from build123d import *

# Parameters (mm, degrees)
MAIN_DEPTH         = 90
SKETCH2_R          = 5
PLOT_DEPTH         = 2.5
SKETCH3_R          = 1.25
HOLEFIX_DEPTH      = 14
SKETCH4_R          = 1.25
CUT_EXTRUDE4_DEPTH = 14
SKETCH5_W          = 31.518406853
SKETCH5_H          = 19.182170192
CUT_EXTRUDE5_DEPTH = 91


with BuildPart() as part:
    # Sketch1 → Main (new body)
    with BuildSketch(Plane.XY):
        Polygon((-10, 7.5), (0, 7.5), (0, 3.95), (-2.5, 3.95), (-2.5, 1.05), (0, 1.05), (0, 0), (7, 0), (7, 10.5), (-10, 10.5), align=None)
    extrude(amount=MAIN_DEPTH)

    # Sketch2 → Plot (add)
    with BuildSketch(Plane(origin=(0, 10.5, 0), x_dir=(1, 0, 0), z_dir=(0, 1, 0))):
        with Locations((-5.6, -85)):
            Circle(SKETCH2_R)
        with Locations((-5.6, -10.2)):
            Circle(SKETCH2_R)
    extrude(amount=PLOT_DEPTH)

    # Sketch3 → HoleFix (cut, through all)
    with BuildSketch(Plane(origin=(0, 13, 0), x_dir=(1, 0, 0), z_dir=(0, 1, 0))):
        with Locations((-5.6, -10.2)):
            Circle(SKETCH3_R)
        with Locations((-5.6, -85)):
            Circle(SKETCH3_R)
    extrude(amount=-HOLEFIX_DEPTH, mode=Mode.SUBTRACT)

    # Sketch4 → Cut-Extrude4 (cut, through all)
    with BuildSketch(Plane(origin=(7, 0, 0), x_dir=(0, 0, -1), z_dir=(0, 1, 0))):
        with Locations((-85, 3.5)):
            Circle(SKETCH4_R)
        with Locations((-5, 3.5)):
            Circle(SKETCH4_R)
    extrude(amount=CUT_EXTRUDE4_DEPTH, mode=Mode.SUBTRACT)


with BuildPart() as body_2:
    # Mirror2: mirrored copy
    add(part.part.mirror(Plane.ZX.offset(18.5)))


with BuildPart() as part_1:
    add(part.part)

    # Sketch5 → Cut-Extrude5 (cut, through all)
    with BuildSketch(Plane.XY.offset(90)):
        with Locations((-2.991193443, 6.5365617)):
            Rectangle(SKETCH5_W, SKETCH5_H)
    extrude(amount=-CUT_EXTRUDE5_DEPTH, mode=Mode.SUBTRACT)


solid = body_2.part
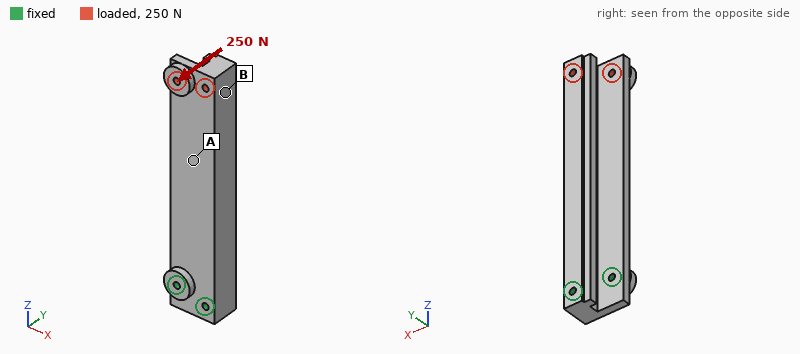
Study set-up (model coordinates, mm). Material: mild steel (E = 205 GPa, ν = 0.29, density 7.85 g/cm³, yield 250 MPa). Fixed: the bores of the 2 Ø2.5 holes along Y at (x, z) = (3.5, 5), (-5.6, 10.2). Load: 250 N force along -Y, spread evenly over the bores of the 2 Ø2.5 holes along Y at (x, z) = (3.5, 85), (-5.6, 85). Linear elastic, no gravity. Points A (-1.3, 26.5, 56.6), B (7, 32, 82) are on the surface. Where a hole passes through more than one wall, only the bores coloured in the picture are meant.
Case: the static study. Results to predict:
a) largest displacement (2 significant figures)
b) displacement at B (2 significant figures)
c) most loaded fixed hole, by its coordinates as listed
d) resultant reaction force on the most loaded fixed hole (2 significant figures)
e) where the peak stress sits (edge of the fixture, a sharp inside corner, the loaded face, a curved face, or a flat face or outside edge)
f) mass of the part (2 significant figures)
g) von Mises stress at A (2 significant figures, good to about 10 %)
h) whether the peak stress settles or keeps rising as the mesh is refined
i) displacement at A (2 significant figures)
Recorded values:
0.27 mm
0.22 mm
(-5.6, 10.2)
620 N
edge of the fixture
80 g
29 MPa
keeps rising
0.12 mm
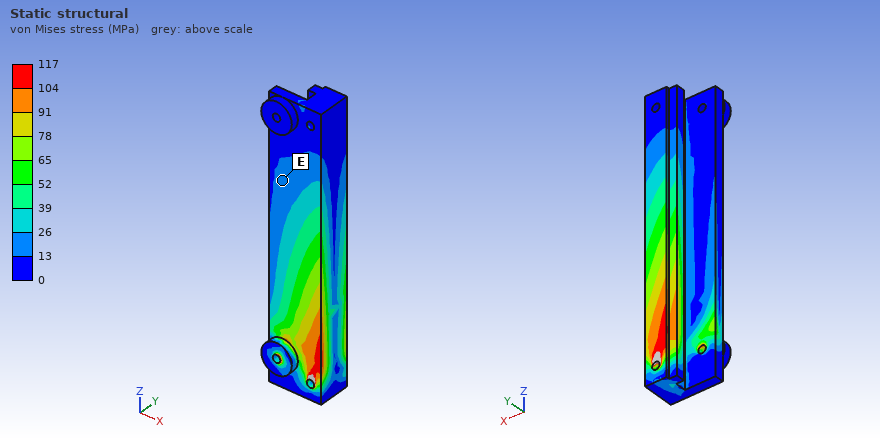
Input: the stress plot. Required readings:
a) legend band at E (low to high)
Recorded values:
13 to 26 MPa
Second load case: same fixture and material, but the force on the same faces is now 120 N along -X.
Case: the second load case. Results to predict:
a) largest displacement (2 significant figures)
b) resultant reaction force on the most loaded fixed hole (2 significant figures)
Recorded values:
70 µm
740 N
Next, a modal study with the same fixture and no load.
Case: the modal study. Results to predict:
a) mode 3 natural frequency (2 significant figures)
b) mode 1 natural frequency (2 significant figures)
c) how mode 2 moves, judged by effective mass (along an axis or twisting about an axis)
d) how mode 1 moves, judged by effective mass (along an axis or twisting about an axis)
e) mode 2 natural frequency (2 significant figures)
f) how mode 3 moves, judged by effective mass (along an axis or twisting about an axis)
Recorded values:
5000 Hz
1000 Hz
along X
along Y
1900 Hz
twisting about Z
